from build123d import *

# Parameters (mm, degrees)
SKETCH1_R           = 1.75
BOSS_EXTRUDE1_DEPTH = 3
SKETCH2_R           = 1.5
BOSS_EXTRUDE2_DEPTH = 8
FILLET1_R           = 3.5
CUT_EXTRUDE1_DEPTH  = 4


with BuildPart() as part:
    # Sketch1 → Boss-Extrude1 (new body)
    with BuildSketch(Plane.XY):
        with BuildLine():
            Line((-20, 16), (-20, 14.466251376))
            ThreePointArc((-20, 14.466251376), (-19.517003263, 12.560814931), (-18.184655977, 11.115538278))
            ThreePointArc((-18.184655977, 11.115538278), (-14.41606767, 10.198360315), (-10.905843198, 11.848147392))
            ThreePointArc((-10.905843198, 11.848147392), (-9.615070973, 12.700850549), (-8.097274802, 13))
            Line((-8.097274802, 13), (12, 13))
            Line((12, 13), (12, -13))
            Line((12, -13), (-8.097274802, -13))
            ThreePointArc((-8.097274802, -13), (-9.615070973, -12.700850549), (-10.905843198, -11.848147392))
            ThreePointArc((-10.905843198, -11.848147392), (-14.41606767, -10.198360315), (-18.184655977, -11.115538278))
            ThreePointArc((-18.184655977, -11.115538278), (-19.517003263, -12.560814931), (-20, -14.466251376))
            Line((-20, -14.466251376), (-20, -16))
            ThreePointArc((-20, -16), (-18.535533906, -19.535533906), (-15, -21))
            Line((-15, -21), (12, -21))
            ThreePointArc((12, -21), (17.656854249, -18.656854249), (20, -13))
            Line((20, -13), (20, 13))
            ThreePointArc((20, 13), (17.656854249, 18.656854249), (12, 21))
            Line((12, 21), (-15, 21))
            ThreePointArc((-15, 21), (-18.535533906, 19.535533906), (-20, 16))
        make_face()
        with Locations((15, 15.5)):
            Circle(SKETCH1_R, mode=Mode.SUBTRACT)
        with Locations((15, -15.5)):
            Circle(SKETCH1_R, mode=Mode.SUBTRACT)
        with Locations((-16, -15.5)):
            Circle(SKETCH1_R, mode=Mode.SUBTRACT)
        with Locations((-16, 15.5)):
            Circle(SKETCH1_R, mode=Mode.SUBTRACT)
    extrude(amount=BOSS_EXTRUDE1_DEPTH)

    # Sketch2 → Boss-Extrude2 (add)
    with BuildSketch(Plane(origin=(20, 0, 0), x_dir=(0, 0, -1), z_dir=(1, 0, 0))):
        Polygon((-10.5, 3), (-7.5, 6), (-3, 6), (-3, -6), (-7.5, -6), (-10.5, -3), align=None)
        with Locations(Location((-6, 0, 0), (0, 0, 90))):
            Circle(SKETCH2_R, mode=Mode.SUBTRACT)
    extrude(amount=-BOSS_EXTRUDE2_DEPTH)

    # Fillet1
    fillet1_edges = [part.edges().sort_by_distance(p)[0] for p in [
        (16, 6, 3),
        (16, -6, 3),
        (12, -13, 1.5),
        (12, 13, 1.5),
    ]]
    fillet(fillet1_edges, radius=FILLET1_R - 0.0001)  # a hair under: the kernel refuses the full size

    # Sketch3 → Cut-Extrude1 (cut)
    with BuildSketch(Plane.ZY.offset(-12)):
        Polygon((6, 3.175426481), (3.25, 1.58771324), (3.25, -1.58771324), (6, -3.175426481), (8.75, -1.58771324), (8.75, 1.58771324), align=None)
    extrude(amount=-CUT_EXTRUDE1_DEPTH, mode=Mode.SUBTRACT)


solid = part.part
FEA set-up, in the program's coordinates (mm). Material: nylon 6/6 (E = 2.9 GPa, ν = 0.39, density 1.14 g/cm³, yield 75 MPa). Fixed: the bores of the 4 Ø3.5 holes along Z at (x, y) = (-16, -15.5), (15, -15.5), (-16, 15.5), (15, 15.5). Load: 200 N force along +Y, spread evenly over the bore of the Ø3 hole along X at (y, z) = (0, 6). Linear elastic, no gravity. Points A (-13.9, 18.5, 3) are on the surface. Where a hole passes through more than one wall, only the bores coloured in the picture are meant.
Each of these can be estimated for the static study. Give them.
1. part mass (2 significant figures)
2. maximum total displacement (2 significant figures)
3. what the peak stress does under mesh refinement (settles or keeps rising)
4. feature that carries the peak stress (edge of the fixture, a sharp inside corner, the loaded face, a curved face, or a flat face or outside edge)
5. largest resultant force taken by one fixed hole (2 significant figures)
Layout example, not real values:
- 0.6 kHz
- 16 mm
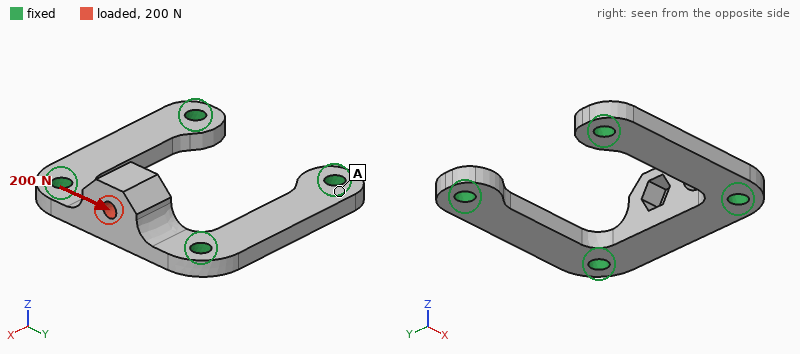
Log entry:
- 3.4 g
- 60 µm
- keeps rising
- edge of the fixture
- 110 N
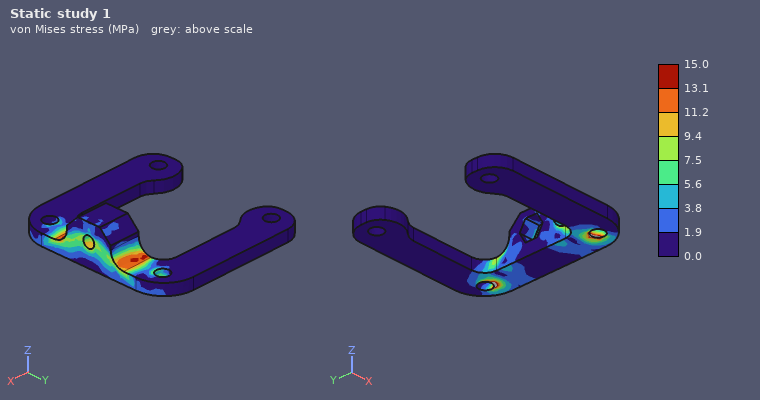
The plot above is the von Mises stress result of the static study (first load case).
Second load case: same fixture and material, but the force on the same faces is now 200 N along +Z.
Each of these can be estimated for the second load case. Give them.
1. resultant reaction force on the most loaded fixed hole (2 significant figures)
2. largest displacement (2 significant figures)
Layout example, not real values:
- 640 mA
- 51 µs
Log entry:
- 120 N
- 0.36 mm
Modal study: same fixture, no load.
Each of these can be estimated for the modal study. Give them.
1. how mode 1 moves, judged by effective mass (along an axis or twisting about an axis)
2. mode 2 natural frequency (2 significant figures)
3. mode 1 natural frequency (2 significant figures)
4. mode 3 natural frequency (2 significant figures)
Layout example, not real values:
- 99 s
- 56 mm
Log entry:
- along X
- 5600 Hz
- 4000 Hz
- 5600 Hz
